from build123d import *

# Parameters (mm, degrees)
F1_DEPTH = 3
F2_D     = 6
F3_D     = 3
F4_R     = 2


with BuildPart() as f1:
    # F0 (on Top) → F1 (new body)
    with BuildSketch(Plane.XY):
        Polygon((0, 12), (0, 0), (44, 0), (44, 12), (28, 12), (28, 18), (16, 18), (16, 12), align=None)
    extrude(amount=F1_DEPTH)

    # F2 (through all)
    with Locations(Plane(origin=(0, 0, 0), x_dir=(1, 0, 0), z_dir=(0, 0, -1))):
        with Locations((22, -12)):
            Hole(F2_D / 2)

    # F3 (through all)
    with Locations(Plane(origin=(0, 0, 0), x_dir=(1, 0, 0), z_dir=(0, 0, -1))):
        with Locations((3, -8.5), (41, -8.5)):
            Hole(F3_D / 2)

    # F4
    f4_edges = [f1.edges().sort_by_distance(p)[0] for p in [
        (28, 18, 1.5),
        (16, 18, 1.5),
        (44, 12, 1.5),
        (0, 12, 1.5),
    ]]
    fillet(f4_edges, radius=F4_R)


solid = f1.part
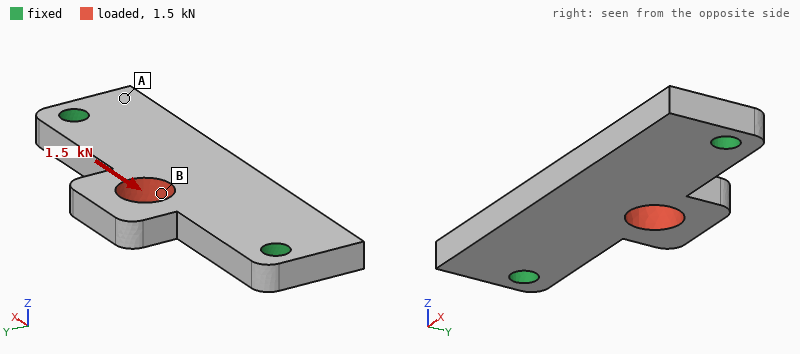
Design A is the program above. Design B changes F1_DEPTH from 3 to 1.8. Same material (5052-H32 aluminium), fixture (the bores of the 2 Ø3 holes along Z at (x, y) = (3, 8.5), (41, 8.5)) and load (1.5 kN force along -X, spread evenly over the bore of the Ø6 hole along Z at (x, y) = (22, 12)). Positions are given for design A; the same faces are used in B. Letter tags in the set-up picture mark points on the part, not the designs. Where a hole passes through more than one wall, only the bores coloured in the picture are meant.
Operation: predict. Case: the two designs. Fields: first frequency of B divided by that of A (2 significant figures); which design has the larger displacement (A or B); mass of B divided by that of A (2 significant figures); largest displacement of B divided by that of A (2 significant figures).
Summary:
0.64
B
0.60
1.7
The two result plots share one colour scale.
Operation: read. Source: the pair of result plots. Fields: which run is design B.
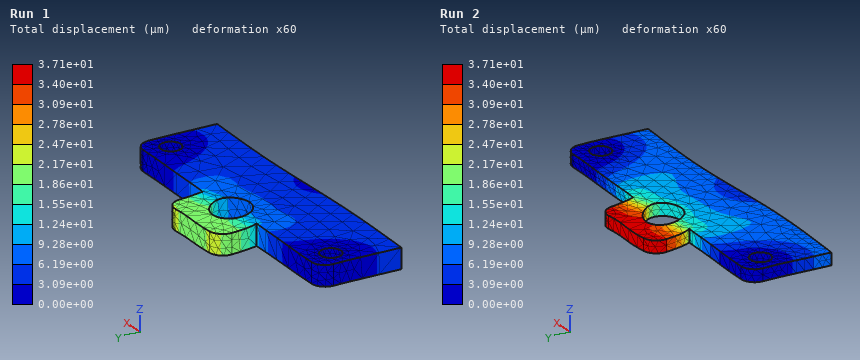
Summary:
Run 2
